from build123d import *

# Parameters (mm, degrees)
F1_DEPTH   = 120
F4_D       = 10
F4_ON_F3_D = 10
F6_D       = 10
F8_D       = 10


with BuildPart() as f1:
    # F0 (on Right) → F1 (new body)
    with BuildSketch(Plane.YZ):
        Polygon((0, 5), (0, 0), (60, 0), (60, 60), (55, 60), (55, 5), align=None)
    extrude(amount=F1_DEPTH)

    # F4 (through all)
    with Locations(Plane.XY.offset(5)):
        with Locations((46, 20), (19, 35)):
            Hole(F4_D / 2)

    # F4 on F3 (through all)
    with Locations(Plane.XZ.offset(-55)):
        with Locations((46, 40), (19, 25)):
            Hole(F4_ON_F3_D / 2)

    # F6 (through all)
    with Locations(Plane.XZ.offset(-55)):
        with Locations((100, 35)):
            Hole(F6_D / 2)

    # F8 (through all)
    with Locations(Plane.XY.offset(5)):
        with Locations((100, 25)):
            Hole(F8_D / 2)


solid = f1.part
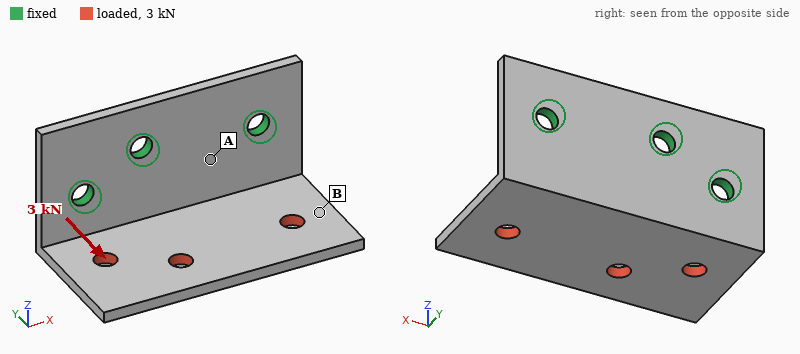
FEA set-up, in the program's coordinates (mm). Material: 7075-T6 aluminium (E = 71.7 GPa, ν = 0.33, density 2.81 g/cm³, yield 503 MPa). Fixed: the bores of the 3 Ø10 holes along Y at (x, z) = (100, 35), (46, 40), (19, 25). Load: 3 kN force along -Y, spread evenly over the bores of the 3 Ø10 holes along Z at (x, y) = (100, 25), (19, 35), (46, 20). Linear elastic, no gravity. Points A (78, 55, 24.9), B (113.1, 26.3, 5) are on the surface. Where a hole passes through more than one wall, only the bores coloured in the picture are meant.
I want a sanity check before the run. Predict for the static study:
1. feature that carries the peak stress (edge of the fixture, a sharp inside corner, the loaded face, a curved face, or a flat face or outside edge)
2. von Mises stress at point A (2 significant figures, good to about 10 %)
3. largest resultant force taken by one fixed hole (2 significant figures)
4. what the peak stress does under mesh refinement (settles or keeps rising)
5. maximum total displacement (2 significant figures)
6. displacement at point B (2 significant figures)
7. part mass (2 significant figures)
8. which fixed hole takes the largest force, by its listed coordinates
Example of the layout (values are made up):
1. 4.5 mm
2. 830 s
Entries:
1. edge of the fixture
2. 63 MPa
3. 1.8 kN
4. keeps rising
5. 0.79 mm
6. 0.48 mm
7. 190 g
8. (19, 25)
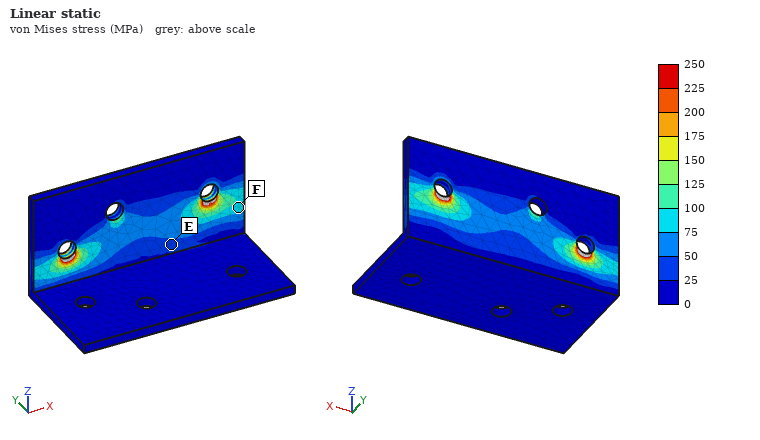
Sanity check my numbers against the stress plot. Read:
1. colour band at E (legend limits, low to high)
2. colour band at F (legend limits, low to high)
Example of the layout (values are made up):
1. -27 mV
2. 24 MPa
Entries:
1. 25 to 50 MPa
2. 75 to 100 MPa
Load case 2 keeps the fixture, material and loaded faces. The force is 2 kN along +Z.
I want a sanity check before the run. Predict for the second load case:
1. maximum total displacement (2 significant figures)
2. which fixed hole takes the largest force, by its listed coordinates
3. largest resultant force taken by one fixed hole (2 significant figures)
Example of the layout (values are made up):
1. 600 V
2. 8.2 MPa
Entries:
1. 1.5 mm
2. (46, 40)
3. 980 N
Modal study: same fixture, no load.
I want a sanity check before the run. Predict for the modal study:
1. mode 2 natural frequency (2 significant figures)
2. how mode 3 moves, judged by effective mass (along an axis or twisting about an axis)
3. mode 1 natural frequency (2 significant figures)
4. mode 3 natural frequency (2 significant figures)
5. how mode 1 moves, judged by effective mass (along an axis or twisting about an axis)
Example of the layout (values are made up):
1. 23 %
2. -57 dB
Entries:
1. 1300 Hz
2. along Y
3. 740 Hz
4. 2100 Hz
5. along Z
